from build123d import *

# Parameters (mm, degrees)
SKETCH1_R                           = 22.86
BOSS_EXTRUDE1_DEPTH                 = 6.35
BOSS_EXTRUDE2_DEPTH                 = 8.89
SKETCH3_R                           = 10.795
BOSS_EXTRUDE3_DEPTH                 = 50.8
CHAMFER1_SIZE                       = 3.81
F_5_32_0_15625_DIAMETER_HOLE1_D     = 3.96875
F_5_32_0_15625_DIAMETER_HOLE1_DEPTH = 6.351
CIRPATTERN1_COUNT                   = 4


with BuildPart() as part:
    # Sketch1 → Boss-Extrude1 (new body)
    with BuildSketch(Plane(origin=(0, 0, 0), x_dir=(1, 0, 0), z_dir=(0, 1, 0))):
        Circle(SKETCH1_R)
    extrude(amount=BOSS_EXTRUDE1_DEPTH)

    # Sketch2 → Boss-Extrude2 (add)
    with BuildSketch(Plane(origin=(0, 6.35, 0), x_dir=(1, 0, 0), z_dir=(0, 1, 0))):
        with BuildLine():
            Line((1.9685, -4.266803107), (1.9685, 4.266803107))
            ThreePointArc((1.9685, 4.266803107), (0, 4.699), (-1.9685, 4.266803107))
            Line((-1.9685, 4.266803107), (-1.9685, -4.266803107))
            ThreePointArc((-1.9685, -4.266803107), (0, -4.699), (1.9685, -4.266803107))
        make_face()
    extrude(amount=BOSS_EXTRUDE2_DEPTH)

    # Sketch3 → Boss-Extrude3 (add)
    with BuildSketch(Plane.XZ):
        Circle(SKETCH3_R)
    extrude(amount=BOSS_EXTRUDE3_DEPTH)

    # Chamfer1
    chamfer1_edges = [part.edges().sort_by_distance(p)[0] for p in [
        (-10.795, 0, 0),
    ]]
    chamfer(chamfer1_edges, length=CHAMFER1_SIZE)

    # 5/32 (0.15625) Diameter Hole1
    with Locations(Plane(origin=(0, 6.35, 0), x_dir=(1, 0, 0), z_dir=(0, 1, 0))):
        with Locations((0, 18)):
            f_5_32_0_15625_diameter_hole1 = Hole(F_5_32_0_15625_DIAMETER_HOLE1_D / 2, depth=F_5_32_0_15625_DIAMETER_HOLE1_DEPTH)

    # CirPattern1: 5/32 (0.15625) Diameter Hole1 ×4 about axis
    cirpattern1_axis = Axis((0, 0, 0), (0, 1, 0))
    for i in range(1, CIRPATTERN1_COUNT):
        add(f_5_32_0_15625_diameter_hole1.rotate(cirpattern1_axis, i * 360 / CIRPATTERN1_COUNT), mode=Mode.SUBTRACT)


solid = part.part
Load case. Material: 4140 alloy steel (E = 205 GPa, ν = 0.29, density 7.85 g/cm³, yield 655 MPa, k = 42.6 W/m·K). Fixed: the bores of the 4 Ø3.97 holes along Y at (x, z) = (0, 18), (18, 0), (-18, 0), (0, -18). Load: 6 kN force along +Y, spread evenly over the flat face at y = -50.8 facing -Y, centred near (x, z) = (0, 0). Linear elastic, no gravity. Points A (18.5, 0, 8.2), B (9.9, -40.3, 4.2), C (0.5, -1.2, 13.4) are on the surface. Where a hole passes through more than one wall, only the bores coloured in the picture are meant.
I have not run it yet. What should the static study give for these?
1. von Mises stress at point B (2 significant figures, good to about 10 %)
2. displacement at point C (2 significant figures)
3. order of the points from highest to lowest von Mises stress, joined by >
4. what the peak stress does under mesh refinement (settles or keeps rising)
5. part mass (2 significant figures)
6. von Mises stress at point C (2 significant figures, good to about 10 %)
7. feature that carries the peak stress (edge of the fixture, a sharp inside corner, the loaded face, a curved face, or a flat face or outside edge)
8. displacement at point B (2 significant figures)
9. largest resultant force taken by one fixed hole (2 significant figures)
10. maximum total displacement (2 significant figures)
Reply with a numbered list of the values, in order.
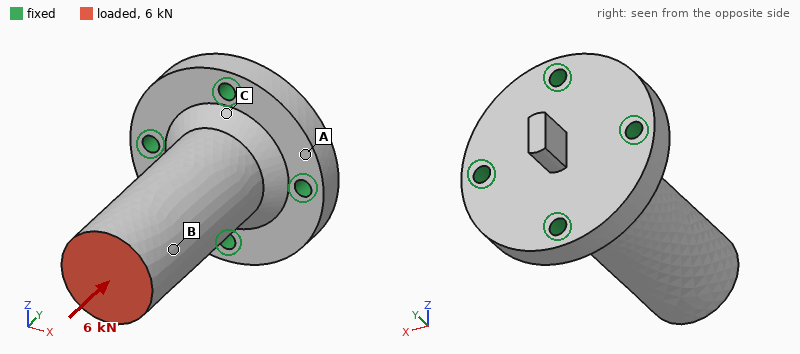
1. 16 MPa
2. 1.6 µm
3. C > B > A
4. keeps rising
5. 230 g
6. 44 MPa
7. edge of the fixture
8. 5.6 µm
9. 1.6 kN
10. 6.5 µm
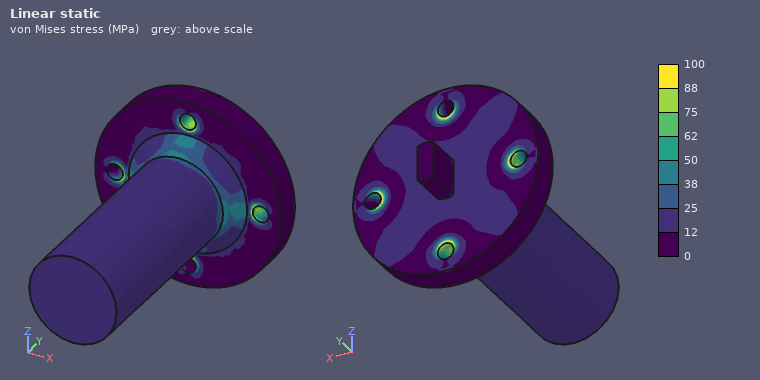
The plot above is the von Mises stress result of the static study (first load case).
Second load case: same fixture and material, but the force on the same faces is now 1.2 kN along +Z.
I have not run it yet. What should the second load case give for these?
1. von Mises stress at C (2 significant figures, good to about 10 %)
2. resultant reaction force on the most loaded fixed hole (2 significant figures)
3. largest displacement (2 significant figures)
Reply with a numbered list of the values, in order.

1. 69 MPa
2. 1.9 kN
3. 37 µm
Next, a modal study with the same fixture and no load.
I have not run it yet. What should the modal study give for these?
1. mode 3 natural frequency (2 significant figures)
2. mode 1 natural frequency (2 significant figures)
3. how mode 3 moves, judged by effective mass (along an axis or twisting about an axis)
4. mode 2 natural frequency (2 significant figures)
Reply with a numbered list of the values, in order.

1. 15 kHz
2. 4500 Hz
3. along Y
4. 4600 Hz
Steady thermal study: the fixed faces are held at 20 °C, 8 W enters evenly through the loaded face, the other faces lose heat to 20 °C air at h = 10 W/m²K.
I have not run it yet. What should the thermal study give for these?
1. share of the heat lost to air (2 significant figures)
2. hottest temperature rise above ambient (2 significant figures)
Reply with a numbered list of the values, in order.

1. 7.6 %
2. 28 K
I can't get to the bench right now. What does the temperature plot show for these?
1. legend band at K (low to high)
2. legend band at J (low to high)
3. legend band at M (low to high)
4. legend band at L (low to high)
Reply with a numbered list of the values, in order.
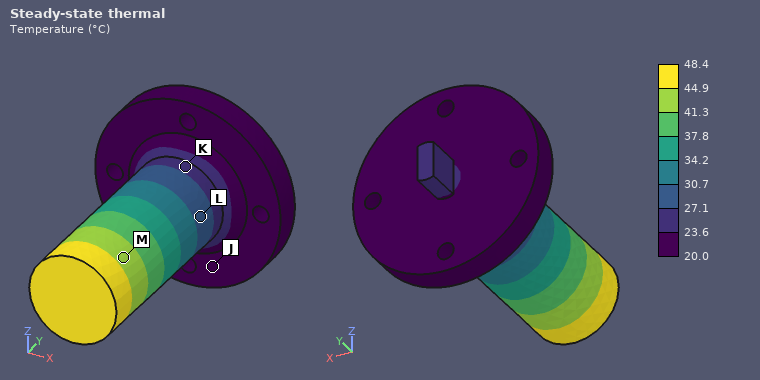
1. 23.6 to 27.1 °C
2. 20.0 to 23.6 °C
3. 41.3 to 44.9 °C
4. 27.1 to 30.7 °C
